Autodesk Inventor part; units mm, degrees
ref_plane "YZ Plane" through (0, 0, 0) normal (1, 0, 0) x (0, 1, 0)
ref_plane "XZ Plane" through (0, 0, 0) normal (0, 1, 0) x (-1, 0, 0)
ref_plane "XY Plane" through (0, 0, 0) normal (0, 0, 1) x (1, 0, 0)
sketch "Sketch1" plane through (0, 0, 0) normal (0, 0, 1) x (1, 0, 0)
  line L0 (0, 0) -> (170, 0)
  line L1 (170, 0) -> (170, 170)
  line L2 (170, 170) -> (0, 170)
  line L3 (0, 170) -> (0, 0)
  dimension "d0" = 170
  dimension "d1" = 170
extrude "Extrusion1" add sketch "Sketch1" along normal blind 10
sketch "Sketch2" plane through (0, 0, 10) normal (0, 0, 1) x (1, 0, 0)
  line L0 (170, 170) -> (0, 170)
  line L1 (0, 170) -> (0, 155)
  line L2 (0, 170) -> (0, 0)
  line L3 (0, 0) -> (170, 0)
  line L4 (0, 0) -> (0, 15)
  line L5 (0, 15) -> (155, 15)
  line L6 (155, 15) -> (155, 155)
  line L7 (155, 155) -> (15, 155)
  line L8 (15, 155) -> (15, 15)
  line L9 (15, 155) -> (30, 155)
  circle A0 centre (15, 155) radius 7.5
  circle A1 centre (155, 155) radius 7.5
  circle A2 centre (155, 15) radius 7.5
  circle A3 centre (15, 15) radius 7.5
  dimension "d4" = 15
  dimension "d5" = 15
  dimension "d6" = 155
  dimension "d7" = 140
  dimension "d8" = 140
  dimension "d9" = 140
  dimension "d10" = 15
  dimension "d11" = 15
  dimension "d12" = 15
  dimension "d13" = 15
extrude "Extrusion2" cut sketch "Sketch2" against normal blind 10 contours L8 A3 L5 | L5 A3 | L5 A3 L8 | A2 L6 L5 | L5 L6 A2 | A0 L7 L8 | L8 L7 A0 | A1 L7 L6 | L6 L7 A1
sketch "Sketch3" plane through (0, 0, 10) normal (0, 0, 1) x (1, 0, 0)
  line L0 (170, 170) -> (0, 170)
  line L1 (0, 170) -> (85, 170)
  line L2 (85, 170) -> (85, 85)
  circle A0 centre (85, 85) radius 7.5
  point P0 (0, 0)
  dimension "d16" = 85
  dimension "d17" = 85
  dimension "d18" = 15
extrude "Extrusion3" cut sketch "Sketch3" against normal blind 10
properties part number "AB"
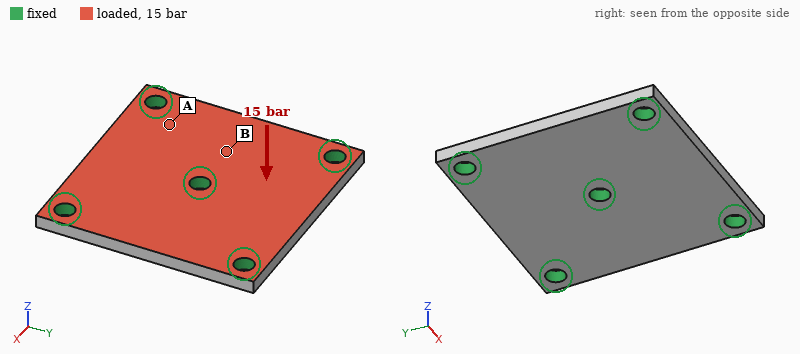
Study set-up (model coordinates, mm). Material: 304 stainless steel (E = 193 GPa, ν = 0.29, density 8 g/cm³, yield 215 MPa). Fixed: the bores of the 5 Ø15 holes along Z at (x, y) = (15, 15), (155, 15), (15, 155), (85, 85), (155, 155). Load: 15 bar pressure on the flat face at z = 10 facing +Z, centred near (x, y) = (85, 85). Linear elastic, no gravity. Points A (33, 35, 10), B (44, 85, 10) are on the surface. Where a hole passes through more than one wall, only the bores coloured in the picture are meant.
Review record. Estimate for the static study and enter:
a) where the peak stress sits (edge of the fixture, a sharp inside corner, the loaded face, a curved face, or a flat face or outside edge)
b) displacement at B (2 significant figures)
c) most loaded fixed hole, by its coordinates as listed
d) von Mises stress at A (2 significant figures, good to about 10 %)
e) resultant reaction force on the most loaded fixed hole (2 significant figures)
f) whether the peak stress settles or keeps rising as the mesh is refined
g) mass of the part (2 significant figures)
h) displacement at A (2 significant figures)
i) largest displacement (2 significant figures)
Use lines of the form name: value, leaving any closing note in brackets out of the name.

where the peak stress sits: edge of the fixture
displacement at B: 32 µm
most loaded fixed hole, by its coordinates as listed: (85, 85)
von Mises stress at A: 44 MPa
resultant reaction force on the most loaded fixed hole: 15 kN
whether the peak stress settles or keeps rising as the mesh is refined: keeps rising
mass of the part: 2.2 kg
displacement at A: 19 µm
largest displacement: 59 µm
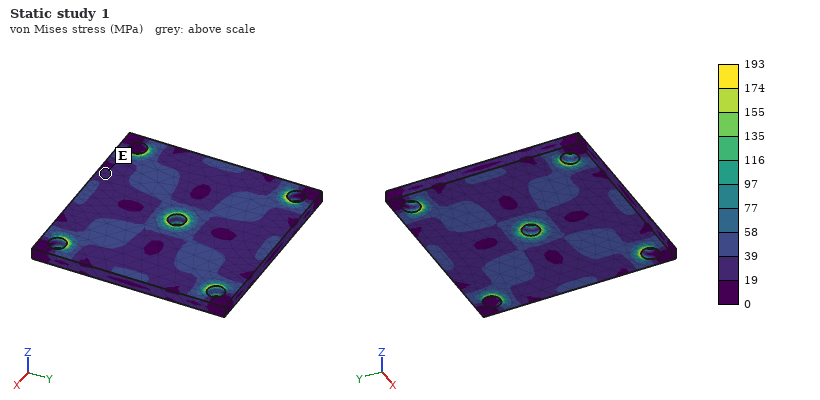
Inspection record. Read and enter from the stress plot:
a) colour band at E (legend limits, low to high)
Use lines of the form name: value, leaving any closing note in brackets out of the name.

colour band at E: 19 to 39 MPa
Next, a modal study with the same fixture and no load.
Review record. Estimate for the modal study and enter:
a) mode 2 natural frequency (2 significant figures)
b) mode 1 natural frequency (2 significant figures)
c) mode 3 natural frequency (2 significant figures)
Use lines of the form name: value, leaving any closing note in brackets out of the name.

mode 2 natural frequency: 3400 Hz
mode 1 natural frequency: 3300 Hz
mode 3 natural frequency: 3400 Hz
